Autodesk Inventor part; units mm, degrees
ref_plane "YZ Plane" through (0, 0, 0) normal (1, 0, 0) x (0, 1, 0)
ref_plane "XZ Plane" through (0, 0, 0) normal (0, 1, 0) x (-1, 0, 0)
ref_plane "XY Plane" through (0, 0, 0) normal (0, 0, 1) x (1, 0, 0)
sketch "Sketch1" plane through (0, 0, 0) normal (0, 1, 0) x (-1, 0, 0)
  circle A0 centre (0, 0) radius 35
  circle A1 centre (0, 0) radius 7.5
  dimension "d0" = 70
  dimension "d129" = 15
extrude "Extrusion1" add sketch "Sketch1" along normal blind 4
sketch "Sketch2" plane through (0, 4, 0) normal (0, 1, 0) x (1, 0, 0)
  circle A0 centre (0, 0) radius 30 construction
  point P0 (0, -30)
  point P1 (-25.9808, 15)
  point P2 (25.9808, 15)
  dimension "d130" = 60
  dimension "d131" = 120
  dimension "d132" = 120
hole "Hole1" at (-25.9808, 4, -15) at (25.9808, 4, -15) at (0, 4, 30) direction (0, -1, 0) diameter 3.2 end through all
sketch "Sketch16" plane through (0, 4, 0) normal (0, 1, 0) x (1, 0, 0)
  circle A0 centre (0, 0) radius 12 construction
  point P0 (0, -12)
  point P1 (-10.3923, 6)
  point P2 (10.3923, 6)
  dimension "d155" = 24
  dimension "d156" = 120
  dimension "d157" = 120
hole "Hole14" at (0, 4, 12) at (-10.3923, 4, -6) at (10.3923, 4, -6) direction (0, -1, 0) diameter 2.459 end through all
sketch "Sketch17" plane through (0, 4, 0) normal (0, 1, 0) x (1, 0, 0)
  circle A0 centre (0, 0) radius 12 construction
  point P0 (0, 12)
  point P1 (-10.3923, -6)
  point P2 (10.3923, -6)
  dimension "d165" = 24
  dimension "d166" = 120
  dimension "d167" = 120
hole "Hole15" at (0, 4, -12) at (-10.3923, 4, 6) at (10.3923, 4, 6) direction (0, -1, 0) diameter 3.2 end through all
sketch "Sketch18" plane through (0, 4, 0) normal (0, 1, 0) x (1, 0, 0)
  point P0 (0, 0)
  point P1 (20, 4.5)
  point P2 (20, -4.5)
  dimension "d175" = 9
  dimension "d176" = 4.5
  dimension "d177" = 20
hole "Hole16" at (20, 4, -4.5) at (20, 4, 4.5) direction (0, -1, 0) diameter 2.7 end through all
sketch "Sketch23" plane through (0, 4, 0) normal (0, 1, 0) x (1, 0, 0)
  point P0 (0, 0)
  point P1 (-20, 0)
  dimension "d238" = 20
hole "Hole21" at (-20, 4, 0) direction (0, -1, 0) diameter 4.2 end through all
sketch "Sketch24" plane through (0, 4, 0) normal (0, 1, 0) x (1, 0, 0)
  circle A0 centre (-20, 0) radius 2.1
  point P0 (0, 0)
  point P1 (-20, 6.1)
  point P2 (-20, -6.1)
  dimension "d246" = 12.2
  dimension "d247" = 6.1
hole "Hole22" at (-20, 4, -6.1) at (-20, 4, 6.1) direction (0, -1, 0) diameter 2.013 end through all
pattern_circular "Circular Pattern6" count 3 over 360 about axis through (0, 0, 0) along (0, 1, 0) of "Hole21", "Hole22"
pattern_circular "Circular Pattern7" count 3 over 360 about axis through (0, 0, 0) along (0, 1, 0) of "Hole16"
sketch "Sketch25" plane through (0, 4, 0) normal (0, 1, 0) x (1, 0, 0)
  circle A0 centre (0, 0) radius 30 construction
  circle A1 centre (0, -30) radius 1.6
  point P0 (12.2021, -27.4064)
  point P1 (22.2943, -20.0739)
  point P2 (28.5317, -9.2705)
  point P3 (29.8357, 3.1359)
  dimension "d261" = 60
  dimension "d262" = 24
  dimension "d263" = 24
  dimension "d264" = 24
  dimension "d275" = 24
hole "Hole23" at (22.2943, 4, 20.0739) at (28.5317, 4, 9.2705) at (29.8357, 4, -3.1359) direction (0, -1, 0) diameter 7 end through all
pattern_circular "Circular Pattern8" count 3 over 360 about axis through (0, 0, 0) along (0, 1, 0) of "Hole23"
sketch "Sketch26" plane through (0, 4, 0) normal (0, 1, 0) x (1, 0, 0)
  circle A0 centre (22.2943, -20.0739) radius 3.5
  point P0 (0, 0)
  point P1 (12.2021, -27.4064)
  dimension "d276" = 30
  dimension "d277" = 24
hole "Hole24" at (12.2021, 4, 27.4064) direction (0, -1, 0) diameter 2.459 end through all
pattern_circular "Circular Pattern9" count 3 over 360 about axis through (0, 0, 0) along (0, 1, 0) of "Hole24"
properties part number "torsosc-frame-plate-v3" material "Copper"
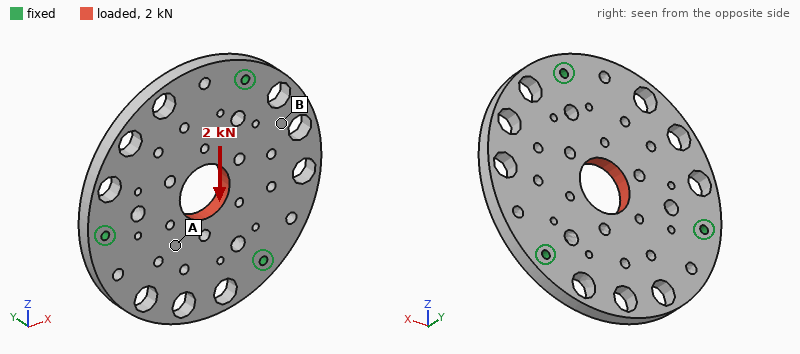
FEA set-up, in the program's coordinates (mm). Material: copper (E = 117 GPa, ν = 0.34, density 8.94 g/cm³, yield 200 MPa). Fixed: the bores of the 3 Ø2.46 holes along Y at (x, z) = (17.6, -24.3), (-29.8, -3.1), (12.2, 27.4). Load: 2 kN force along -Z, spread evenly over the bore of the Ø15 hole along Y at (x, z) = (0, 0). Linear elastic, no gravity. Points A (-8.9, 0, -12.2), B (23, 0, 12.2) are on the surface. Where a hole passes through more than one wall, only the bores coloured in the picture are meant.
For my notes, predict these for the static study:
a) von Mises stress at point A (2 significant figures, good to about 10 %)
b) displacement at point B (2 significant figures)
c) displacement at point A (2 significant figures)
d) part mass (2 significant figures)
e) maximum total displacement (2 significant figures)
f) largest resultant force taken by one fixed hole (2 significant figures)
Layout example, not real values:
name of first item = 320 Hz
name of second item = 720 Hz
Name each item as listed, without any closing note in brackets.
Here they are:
von Mises stress at point A = 6.8 MPa
displacement at point B = 1.5 µm
displacement at point A = 4.1 µm
part mass = 110 g
maximum total displacement = 4.9 µm
largest resultant force taken by one fixed hole = 720 N
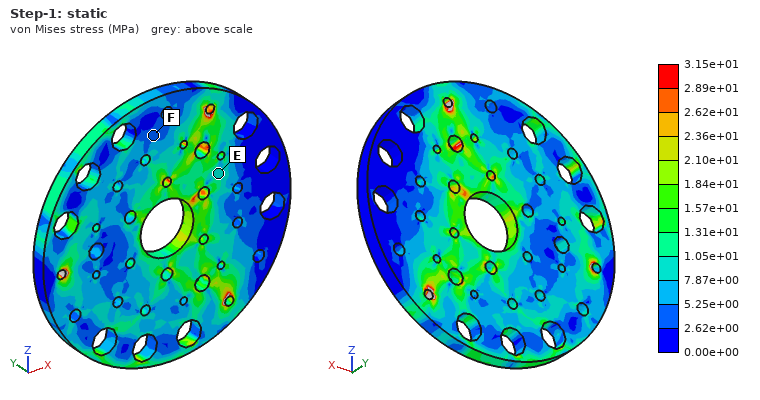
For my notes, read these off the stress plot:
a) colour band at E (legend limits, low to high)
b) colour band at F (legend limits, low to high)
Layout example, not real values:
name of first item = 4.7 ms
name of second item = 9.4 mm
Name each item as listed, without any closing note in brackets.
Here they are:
colour band at E = 7.87e+00 to 1.05e+01 MPa
colour band at F = 2.62e+00 to 5.25e+00 MPa
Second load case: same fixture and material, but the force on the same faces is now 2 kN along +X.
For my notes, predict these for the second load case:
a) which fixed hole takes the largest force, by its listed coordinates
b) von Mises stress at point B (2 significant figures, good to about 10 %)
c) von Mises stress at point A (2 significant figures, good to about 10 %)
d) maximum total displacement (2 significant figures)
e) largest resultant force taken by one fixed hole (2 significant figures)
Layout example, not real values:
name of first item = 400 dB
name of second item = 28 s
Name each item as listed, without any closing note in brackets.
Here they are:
which fixed hole takes the largest force, by its listed coordinates = (-29.8, -3.1)
von Mises stress at point B = 8.7 MPa
von Mises stress at point A = 8.1 MPa
maximum total displacement = 5.1 µm
largest resultant force taken by one fixed hole = 750 N
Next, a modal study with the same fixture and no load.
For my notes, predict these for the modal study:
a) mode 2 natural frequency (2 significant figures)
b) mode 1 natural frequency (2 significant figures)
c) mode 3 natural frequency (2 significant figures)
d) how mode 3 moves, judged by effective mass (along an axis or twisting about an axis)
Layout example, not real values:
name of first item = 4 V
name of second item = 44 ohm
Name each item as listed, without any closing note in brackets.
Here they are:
mode 2 natural frequency = 3500 Hz
mode 1 natural frequency = 3500 Hz
mode 3 natural frequency = 4000 Hz
how mode 3 moves, judged by effective mass = along Y
